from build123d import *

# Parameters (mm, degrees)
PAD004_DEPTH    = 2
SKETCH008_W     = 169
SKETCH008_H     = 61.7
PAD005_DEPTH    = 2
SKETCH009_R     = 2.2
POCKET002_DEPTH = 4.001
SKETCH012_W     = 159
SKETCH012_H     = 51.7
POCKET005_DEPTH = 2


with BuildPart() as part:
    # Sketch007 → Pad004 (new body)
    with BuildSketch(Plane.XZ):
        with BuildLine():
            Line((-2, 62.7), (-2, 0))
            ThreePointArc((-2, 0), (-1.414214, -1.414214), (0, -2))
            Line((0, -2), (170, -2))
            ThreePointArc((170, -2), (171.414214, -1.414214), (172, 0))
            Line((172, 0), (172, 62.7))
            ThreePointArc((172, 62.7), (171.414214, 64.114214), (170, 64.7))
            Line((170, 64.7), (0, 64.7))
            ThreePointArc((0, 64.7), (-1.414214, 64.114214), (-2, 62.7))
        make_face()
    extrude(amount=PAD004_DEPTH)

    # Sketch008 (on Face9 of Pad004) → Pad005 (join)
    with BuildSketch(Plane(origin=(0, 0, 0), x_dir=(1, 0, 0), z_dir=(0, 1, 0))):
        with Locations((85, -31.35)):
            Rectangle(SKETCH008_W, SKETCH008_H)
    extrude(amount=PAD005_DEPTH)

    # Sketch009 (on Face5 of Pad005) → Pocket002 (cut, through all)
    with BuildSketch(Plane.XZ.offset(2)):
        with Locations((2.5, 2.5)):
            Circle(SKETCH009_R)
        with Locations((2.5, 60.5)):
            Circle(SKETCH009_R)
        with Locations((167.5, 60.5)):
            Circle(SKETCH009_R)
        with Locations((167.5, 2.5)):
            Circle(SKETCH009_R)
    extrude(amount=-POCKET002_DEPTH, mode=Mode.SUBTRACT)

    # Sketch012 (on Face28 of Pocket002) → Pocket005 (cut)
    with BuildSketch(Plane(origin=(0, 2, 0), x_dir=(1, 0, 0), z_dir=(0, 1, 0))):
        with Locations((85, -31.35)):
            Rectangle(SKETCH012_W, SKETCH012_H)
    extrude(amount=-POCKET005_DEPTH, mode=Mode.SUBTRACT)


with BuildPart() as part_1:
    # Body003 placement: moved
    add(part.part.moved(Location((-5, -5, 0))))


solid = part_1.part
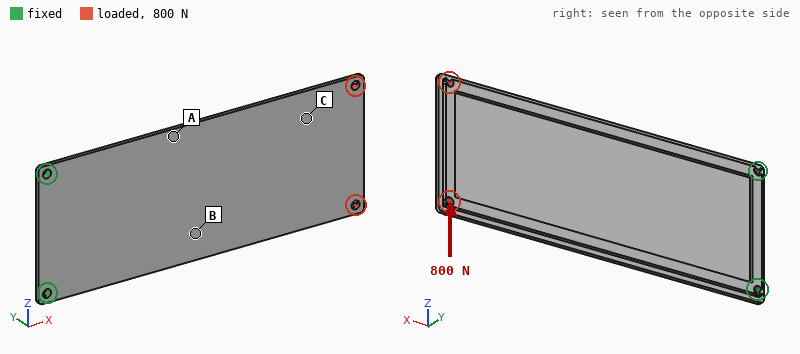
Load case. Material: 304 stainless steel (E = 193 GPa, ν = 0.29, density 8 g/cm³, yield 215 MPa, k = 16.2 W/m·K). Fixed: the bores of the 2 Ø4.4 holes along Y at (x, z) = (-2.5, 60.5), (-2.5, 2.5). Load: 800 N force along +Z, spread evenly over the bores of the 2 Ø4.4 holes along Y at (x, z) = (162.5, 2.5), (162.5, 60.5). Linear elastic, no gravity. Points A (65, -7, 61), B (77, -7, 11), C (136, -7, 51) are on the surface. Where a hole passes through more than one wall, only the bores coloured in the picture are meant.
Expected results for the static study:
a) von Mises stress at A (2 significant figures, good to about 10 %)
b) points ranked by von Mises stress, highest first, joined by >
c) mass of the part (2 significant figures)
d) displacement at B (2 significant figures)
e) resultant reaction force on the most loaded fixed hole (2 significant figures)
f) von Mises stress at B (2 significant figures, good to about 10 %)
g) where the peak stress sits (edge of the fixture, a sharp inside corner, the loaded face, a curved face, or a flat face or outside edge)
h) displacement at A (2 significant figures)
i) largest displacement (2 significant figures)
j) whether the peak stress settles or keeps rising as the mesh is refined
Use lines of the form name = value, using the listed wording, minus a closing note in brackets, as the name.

von Mises stress at A = 38 MPa
points ranked by von Mises stress, highest first, joined by > = A > B > C
mass of the part = 220 g
displacement at B = 0.066 mm
resultant reaction force on the most loaded fixed hole = 2.3 kN
von Mises stress at B = 22 MPa
where the peak stress sits = a sharp inside corner
displacement at A = 0.075 mm
largest displacement = 0.25 mm
whether the peak stress settles or keeps rising as the mesh is refined = keeps rising
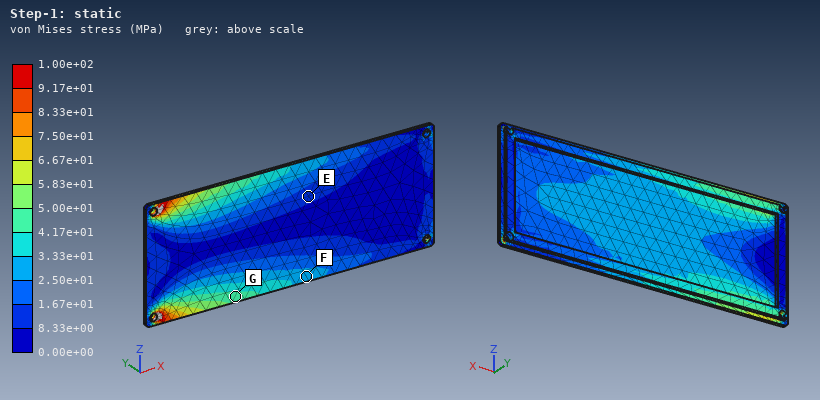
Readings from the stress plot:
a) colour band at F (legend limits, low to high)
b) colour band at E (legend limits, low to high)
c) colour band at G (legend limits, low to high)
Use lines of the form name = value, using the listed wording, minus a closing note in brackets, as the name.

colour band at F = 2.50e+01 to 3.33e+01 MPa
colour band at E = 8.33e+00 to 1.67e+01 MPa
colour band at G = 4.17e+01 to 5.00e+01 MPa
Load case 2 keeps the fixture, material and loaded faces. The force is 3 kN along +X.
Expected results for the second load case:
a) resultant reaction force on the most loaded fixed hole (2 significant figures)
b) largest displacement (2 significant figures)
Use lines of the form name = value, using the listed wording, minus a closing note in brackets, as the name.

resultant reaction force on the most loaded fixed hole = 1.6 kN
largest displacement = 0.89 mm
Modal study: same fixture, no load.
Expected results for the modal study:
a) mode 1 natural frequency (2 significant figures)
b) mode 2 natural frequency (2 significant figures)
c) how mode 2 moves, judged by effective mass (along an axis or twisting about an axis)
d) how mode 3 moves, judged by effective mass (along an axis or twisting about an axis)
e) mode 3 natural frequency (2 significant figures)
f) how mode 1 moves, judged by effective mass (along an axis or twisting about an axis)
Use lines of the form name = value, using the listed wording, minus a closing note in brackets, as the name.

mode 1 natural frequency = 82 Hz
mode 2 natural frequency = 360 Hz
how mode 2 moves, judged by effective mass = twisting about X
how mode 3 moves, judged by effective mass = along Y
mode 3 natural frequency = 520 Hz
how mode 1 moves, judged by effective mass = along Y
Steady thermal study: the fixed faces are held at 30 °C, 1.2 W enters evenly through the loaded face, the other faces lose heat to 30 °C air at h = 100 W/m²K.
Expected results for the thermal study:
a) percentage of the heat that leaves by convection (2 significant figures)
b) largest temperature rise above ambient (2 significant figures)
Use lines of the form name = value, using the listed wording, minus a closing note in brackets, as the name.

percentage of the heat that leaves by convection = 100 %
largest temperature rise above ambient = 18 K
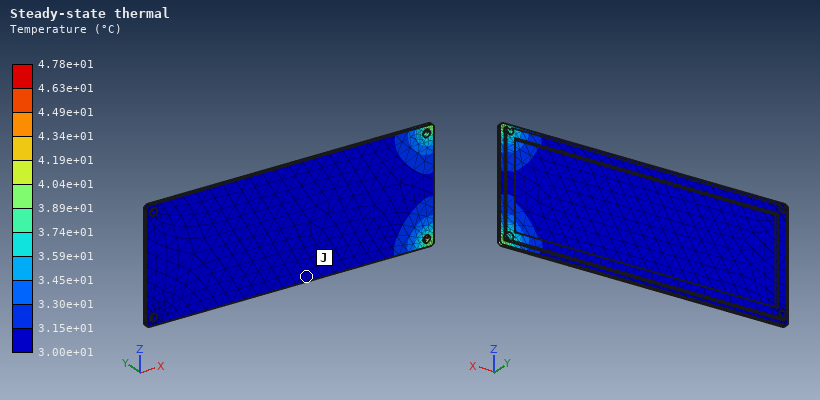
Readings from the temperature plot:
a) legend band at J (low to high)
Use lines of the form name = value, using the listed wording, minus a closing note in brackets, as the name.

legend band at J = 3.00e+01 to 3.15e+01 °C
